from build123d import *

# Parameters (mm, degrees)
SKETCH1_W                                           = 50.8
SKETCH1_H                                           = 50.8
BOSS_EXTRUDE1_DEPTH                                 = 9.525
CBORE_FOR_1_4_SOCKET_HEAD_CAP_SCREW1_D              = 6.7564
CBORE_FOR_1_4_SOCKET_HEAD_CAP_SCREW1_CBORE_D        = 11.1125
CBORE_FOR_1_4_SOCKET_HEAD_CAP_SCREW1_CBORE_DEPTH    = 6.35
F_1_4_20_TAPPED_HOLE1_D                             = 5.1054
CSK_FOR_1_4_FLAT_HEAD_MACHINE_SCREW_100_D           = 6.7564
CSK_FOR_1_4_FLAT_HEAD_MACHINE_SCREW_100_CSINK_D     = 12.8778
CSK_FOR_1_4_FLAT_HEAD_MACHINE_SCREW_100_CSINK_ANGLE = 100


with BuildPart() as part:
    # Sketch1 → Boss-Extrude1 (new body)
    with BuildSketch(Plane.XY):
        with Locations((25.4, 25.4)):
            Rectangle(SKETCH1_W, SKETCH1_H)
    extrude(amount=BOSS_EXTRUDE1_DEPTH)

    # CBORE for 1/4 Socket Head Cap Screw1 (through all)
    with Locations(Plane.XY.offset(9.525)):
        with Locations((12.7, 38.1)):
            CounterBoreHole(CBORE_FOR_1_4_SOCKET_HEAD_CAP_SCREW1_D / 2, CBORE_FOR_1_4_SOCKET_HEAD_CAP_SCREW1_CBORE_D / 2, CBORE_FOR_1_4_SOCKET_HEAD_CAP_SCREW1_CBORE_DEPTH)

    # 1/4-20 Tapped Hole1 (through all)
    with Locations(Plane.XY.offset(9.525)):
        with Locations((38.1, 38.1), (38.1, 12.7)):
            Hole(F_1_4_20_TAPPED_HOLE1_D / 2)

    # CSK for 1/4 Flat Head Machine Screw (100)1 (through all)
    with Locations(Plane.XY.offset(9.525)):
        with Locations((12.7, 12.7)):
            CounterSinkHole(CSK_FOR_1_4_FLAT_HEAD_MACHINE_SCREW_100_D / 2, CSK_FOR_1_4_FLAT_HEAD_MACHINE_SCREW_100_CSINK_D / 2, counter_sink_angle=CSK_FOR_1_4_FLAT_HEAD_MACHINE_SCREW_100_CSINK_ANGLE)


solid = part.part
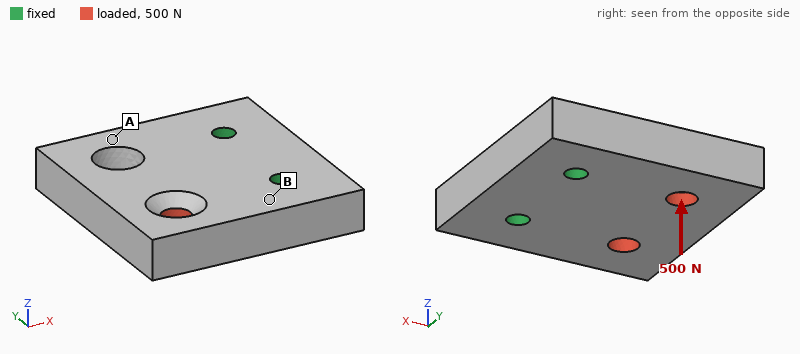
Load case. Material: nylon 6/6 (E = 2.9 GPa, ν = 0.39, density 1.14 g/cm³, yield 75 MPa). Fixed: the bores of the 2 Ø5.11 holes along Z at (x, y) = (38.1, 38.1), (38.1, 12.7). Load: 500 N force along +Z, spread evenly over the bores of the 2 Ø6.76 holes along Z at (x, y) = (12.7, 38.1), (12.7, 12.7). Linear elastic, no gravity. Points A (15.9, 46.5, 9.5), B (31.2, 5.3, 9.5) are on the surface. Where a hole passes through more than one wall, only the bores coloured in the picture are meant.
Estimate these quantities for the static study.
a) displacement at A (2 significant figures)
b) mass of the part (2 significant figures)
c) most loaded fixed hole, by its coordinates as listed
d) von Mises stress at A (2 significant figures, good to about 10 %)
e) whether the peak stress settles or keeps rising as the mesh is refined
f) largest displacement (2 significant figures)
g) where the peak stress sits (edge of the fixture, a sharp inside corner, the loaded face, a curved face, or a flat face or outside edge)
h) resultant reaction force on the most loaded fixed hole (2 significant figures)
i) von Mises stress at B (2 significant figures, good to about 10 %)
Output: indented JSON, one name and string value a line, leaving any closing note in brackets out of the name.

{
  "displacement at A": "0.21 mm",
  "mass of the part": "26 g",
  "most loaded fixed hole, by its coordinates as listed": "(38.1, 12.7)",
  "von Mises stress at A": "4.4 MPa",
  "whether the peak stress settles or keeps rising as the mesh is refined": "keeps rising",
  "largest displacement": "0.59 mm",
  "where the peak stress sits": "edge of the fixture",
  "resultant reaction force on the most loaded fixed hole": "320 N",
  "von Mises stress at B": "11 MPa"
}
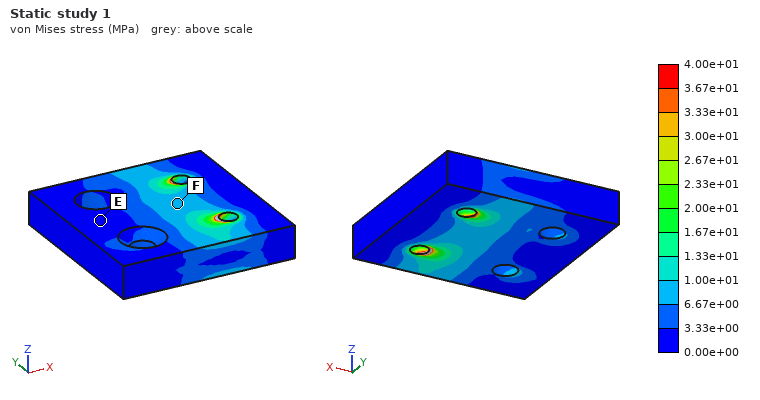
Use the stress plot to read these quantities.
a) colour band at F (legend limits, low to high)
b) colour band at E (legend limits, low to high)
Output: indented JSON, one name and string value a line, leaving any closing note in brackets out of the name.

{
  "colour band at F": "6.67e+00 to 1.00e+01 MPa",
  "colour band at E": "0.00e+00 to 3.33e+00 MPa"
}
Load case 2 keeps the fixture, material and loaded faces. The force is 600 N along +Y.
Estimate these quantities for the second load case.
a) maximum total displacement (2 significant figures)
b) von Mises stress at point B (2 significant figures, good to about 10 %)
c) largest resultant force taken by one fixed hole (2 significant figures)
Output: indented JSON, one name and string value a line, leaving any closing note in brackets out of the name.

{
  "maximum total displacement": "0.10 mm",
  "von Mises stress at point B": "2.1 MPa",
  "largest resultant force taken by one fixed hole": "600 N"
}
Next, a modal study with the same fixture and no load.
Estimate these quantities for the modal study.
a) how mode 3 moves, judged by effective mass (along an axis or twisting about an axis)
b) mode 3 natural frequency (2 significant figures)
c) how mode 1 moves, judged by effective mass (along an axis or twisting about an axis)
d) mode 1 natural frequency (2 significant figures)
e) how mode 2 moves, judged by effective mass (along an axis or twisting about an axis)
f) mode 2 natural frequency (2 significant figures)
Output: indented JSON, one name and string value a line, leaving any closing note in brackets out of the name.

{
  "how mode 3 moves, judged by effective mass": "along Y",
  "mode 3 natural frequency": "3900 Hz",
  "how mode 1 moves, judged by effective mass": "along Z",
  "mode 1 natural frequency": "1600 Hz",
  "how mode 2 moves, judged by effective mass": "twisting about X",
  "mode 2 natural frequency": "2700 Hz"
}
